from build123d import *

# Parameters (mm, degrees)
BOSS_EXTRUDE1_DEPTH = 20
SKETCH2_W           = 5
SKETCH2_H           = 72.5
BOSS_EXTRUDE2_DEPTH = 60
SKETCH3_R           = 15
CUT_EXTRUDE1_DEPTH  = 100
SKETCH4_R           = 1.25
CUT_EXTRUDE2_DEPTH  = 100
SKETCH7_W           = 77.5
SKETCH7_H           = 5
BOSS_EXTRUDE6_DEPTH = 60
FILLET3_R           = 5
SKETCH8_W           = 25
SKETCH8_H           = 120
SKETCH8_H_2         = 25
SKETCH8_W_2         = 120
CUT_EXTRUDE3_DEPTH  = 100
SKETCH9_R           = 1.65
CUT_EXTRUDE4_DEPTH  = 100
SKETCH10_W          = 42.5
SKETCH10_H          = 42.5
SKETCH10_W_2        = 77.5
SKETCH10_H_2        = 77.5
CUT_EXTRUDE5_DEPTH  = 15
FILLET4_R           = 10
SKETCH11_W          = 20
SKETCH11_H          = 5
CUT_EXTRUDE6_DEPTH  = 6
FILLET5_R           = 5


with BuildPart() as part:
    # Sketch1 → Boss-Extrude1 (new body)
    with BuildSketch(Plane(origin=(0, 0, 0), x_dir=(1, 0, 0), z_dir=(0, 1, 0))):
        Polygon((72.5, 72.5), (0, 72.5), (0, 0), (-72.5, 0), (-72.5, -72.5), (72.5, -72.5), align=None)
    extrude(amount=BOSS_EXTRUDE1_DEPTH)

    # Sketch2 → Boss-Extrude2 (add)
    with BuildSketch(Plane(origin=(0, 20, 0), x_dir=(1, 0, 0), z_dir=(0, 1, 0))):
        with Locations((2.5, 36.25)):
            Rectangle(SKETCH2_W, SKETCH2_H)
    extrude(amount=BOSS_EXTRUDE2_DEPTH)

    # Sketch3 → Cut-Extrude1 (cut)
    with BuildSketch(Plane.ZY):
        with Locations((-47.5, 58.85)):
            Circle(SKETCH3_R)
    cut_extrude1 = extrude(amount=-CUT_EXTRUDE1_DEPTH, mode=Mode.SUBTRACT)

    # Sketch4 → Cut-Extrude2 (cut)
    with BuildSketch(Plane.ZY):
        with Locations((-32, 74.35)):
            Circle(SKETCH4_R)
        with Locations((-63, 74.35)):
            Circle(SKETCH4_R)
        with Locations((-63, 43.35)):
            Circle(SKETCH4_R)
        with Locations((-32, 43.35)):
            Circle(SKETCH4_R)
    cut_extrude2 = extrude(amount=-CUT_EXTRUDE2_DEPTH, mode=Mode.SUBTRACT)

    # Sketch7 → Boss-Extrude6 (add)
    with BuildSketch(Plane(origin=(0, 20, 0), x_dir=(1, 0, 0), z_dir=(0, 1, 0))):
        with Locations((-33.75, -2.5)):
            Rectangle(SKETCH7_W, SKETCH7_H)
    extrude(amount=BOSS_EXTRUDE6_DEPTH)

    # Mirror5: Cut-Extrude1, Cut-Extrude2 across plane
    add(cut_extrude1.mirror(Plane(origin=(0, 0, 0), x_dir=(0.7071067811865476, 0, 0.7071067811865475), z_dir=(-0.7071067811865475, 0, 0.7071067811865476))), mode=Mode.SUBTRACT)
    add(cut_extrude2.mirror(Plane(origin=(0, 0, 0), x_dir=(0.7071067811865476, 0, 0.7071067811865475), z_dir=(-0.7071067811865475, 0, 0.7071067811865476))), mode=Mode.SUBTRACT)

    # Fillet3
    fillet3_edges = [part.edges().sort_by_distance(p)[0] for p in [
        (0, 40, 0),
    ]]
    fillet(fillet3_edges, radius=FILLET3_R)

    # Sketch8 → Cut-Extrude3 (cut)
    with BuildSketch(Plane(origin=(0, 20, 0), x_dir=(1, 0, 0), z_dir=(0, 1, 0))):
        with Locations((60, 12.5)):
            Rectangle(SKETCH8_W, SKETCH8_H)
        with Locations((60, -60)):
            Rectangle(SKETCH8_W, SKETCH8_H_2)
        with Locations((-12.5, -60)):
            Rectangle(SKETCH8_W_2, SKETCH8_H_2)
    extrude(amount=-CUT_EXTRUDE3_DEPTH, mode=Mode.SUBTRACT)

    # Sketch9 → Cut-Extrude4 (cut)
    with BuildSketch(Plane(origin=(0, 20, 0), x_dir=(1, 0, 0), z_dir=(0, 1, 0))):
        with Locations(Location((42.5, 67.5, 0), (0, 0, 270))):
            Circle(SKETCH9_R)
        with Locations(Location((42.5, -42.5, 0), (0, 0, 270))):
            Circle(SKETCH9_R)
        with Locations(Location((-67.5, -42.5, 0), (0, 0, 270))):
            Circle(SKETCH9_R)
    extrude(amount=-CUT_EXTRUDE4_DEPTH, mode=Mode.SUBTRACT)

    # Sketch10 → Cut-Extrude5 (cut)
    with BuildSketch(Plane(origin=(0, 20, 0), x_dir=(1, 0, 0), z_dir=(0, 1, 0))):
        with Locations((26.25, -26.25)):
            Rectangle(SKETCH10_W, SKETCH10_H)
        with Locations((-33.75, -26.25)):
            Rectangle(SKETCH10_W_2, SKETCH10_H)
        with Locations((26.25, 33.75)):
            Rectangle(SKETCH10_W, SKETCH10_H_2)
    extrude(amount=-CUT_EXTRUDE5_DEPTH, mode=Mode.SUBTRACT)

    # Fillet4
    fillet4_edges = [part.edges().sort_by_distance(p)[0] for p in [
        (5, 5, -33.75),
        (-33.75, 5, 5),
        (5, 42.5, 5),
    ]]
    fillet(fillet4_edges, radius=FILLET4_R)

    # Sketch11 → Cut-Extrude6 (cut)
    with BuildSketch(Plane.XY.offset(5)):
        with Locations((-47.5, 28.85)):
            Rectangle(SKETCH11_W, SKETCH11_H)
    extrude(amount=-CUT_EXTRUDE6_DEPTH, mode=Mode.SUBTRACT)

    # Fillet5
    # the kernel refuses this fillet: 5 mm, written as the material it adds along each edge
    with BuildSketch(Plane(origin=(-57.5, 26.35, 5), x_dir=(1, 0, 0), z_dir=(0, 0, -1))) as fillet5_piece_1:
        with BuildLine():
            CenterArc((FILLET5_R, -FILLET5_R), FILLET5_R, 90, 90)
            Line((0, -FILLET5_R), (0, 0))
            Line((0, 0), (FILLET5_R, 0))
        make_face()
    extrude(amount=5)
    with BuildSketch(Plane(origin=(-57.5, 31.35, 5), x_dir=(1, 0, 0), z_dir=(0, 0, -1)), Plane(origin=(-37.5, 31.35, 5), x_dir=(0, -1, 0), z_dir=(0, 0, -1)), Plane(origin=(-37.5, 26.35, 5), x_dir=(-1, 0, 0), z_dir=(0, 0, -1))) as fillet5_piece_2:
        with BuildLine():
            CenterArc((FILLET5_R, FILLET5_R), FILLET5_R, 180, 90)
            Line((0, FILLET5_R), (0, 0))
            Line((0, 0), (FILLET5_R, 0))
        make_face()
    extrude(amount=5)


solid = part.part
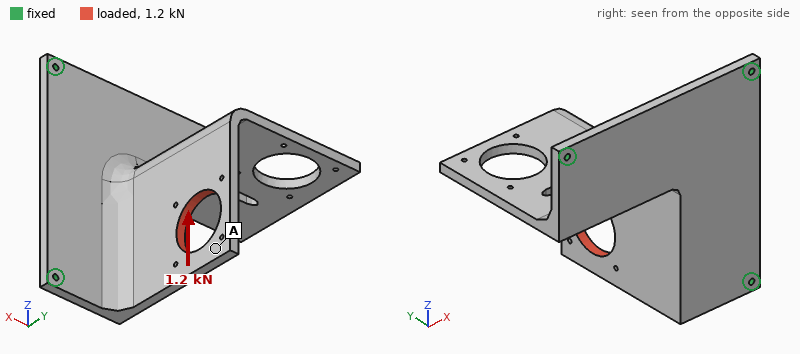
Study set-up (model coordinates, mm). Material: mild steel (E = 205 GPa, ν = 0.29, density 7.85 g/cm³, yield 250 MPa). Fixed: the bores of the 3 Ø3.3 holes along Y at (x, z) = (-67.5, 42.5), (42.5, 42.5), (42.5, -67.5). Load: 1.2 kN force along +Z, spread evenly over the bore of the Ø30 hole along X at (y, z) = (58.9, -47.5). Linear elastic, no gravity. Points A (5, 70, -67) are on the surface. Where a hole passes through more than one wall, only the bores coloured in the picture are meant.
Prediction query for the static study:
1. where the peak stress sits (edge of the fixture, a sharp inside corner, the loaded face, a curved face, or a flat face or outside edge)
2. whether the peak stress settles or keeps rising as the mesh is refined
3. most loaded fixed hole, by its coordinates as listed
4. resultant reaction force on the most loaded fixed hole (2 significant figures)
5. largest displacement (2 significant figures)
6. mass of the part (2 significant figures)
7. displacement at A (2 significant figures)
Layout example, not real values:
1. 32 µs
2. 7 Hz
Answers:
1. edge of the fixture
2. keeps rising
3. (42.5, 42.5)
4. 900 N
5. 0.28 mm
6. 760 g
7. 0.25 mm
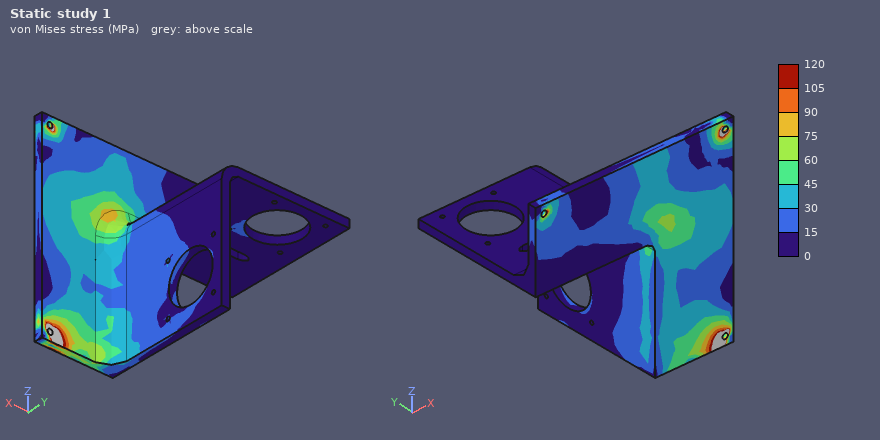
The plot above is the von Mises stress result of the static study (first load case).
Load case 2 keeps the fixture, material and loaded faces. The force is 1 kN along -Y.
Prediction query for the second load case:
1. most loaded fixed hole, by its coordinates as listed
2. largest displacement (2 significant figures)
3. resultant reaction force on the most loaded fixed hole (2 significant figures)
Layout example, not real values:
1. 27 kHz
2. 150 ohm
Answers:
1. (42.5, -67.5)
2. 0.20 mm
3. 850 N
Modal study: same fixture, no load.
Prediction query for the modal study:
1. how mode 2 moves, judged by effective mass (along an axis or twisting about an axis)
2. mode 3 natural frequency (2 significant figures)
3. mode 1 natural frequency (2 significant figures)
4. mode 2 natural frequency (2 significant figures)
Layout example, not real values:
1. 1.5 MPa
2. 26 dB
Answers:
1. along Y
2. 1100 Hz
3. 690 Hz
4. 1100 Hz
